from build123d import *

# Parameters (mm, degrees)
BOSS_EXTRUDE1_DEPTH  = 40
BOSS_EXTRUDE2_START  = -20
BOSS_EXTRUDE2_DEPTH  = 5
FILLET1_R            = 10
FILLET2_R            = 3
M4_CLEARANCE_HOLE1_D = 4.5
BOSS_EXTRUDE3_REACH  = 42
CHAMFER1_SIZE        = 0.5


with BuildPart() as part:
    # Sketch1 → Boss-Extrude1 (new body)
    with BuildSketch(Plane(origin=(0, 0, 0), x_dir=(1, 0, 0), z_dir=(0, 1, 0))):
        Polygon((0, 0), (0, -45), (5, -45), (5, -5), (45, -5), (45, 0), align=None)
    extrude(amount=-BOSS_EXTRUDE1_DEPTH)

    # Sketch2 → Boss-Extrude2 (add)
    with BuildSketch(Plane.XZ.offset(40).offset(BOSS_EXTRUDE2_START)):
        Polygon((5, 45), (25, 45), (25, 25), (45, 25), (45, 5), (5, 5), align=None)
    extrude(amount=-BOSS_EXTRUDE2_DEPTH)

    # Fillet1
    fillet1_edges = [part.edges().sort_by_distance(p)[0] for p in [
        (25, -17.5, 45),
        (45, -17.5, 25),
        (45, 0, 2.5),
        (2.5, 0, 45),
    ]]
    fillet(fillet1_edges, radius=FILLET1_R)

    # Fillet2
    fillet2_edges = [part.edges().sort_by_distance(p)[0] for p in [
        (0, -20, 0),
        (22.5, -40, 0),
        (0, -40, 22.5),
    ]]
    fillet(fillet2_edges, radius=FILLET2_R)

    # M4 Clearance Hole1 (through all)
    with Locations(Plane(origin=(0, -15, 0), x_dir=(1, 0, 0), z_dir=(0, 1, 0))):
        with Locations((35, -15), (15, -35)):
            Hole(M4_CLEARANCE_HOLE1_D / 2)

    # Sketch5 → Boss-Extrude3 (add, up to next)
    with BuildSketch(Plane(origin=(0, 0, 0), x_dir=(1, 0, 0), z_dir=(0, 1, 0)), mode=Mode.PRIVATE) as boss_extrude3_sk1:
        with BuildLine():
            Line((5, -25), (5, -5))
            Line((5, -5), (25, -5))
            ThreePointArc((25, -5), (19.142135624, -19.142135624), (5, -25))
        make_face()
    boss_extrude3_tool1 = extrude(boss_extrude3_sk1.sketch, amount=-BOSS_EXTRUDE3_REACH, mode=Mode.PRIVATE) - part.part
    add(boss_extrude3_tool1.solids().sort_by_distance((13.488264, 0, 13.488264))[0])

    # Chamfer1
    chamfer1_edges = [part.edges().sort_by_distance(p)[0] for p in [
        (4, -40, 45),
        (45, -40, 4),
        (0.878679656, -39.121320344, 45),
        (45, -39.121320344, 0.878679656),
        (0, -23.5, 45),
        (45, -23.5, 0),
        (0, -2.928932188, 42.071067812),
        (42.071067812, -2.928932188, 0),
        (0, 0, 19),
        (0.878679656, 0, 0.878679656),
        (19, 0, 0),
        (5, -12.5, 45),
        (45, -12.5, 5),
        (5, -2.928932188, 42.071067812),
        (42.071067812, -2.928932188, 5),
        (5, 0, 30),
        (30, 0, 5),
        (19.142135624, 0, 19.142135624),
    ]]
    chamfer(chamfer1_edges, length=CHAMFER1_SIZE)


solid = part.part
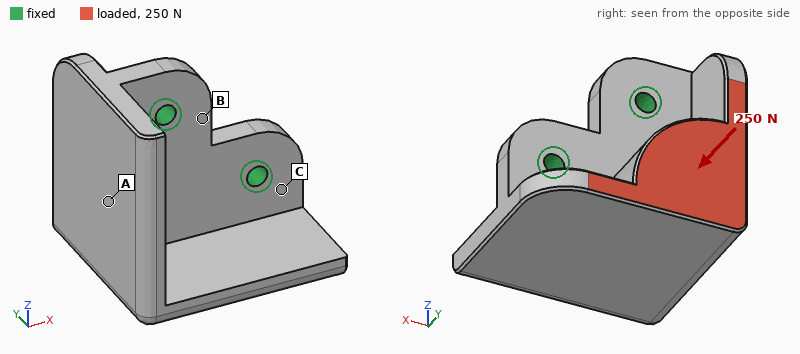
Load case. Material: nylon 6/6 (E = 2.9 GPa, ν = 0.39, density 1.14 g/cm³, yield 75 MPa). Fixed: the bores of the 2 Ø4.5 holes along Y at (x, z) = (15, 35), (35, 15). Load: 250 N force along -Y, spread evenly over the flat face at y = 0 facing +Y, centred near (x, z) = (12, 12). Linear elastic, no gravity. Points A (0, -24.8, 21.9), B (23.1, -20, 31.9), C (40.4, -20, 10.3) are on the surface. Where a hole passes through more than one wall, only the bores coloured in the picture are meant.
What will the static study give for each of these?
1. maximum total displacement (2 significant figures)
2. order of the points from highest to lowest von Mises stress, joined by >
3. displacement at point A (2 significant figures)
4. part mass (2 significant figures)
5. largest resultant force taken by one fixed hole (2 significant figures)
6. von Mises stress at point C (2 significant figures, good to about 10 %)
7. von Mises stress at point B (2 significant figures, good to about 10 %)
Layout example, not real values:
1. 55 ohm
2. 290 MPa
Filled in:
1. 0.77 mm
2. C > B > A
3. 0.37 mm
4. 31 g
5. 130 N
6. 9.5 MPa
7. 5.3 MPa
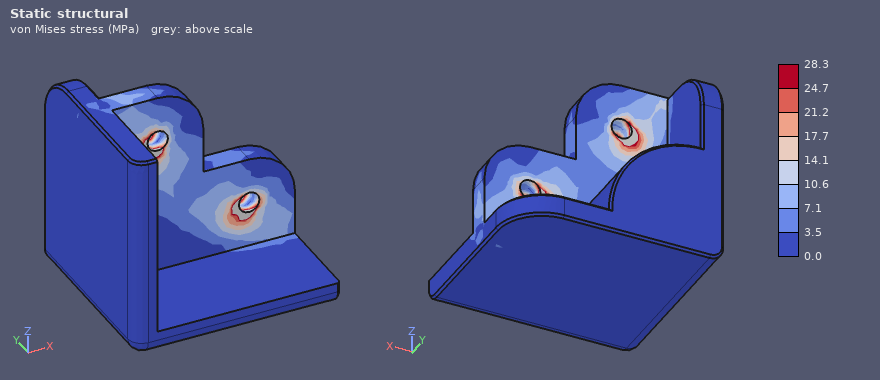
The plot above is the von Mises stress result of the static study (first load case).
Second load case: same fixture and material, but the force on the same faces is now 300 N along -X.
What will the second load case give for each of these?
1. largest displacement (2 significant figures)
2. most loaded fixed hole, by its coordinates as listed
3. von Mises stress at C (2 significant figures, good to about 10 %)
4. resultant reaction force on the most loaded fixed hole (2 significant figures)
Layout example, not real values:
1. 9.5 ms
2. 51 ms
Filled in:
1. 0.79 mm
2. (35, 15)
3. 8.5 MPa
4. 290 N
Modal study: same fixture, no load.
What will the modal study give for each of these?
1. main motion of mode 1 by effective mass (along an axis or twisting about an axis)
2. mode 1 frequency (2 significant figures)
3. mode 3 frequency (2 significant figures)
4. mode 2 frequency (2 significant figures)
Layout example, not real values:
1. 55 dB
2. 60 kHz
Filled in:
1. along Y
2. 700 Hz
3. 2900 Hz
4. 1800 Hz
